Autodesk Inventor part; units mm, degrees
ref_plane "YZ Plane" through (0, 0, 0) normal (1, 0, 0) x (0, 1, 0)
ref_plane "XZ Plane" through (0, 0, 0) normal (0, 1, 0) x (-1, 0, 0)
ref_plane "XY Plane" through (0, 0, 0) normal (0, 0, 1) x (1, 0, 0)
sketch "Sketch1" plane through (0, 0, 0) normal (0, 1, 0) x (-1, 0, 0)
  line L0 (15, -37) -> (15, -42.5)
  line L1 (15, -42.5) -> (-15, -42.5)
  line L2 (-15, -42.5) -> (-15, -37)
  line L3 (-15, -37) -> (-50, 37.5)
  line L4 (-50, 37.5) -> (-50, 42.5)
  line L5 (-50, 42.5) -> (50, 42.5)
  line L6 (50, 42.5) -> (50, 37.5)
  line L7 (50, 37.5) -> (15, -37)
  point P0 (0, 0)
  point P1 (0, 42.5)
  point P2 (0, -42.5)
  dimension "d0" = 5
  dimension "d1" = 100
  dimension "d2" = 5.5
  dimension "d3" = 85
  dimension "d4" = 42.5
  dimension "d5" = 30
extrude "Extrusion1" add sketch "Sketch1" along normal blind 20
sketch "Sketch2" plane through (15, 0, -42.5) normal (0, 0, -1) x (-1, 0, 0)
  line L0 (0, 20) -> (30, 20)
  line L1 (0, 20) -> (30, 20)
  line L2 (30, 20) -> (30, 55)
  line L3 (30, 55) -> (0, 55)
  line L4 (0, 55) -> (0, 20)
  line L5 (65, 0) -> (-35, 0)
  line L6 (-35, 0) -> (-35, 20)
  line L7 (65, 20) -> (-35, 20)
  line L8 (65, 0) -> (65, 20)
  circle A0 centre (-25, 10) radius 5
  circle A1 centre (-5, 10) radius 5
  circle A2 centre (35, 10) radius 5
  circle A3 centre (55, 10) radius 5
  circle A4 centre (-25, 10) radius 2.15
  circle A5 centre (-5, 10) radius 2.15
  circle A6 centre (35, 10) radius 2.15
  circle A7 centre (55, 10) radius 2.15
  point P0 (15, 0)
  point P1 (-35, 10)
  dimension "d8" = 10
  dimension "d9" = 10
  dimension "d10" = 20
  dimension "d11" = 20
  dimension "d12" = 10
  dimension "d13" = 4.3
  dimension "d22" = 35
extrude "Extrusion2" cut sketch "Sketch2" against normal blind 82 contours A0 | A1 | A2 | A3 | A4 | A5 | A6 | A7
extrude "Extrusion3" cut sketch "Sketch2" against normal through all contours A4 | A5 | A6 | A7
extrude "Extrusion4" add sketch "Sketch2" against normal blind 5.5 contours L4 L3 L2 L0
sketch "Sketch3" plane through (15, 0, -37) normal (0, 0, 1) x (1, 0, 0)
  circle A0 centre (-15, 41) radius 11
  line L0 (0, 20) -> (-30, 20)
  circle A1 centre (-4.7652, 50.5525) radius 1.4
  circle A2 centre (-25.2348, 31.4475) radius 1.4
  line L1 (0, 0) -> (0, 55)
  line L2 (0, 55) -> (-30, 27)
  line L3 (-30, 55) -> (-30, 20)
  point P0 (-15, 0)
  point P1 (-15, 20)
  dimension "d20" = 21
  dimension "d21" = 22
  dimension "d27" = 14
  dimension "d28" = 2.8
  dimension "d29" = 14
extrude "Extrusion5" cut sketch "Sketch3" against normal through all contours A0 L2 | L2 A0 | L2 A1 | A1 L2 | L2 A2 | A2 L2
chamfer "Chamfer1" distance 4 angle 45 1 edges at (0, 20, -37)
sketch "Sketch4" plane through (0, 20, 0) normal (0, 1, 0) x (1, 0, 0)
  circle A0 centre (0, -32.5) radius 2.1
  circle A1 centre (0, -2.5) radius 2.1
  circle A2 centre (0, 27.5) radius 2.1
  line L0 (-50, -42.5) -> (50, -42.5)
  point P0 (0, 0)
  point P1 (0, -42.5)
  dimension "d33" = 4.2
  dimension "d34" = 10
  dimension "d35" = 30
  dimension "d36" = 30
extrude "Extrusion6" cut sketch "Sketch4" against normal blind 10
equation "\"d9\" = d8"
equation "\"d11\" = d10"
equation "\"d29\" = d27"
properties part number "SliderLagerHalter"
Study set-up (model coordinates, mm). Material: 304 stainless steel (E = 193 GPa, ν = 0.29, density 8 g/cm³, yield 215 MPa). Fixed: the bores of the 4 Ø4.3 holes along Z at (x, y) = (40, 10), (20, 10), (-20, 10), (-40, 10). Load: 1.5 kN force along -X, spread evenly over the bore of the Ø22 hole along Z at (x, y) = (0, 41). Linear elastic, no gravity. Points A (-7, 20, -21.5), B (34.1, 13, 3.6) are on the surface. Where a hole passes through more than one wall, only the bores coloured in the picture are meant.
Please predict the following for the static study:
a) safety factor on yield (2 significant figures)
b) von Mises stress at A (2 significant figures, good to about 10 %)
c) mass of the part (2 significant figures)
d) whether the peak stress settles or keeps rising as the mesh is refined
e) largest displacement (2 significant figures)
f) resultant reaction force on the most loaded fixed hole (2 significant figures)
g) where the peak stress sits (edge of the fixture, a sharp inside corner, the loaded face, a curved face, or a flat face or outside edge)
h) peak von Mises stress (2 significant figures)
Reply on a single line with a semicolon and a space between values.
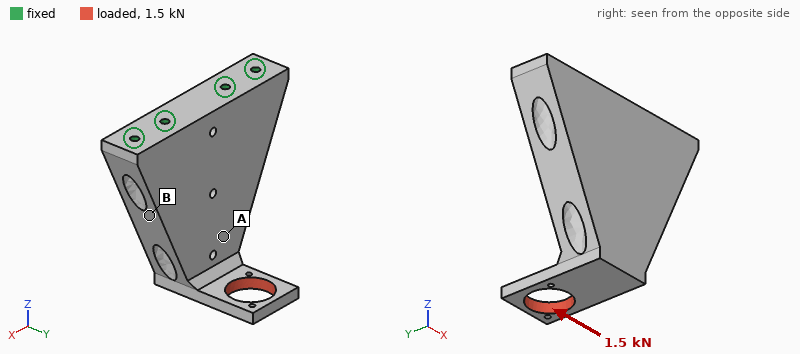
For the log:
1.7; 24 MPa; 800 g; settles; 73 µm; 1.3 kN; the loaded face; 120 MPa
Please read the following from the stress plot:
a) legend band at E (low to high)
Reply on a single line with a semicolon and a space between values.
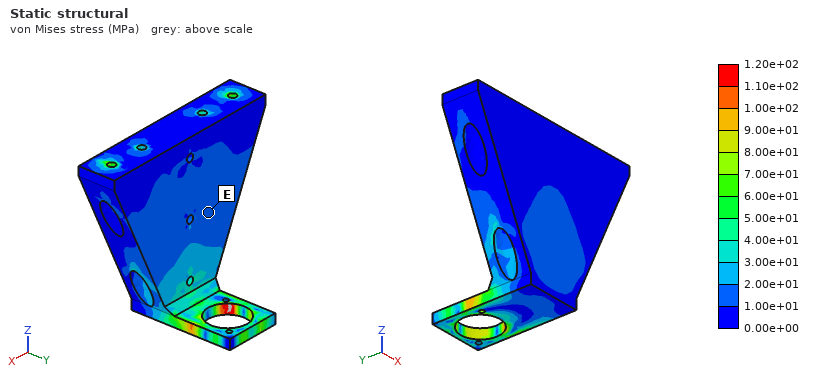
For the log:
1.00e+01 to 2.00e+01 MPa
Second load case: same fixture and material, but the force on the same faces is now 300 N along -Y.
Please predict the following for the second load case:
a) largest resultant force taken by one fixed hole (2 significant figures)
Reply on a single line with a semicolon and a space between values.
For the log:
140 N
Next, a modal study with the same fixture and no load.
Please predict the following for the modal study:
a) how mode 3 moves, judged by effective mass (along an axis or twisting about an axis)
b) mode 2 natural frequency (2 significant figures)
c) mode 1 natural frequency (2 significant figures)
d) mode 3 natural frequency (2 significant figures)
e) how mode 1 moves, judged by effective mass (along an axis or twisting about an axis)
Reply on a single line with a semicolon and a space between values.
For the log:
along X; 3300 Hz; 690 Hz; 4500 Hz; along Y
